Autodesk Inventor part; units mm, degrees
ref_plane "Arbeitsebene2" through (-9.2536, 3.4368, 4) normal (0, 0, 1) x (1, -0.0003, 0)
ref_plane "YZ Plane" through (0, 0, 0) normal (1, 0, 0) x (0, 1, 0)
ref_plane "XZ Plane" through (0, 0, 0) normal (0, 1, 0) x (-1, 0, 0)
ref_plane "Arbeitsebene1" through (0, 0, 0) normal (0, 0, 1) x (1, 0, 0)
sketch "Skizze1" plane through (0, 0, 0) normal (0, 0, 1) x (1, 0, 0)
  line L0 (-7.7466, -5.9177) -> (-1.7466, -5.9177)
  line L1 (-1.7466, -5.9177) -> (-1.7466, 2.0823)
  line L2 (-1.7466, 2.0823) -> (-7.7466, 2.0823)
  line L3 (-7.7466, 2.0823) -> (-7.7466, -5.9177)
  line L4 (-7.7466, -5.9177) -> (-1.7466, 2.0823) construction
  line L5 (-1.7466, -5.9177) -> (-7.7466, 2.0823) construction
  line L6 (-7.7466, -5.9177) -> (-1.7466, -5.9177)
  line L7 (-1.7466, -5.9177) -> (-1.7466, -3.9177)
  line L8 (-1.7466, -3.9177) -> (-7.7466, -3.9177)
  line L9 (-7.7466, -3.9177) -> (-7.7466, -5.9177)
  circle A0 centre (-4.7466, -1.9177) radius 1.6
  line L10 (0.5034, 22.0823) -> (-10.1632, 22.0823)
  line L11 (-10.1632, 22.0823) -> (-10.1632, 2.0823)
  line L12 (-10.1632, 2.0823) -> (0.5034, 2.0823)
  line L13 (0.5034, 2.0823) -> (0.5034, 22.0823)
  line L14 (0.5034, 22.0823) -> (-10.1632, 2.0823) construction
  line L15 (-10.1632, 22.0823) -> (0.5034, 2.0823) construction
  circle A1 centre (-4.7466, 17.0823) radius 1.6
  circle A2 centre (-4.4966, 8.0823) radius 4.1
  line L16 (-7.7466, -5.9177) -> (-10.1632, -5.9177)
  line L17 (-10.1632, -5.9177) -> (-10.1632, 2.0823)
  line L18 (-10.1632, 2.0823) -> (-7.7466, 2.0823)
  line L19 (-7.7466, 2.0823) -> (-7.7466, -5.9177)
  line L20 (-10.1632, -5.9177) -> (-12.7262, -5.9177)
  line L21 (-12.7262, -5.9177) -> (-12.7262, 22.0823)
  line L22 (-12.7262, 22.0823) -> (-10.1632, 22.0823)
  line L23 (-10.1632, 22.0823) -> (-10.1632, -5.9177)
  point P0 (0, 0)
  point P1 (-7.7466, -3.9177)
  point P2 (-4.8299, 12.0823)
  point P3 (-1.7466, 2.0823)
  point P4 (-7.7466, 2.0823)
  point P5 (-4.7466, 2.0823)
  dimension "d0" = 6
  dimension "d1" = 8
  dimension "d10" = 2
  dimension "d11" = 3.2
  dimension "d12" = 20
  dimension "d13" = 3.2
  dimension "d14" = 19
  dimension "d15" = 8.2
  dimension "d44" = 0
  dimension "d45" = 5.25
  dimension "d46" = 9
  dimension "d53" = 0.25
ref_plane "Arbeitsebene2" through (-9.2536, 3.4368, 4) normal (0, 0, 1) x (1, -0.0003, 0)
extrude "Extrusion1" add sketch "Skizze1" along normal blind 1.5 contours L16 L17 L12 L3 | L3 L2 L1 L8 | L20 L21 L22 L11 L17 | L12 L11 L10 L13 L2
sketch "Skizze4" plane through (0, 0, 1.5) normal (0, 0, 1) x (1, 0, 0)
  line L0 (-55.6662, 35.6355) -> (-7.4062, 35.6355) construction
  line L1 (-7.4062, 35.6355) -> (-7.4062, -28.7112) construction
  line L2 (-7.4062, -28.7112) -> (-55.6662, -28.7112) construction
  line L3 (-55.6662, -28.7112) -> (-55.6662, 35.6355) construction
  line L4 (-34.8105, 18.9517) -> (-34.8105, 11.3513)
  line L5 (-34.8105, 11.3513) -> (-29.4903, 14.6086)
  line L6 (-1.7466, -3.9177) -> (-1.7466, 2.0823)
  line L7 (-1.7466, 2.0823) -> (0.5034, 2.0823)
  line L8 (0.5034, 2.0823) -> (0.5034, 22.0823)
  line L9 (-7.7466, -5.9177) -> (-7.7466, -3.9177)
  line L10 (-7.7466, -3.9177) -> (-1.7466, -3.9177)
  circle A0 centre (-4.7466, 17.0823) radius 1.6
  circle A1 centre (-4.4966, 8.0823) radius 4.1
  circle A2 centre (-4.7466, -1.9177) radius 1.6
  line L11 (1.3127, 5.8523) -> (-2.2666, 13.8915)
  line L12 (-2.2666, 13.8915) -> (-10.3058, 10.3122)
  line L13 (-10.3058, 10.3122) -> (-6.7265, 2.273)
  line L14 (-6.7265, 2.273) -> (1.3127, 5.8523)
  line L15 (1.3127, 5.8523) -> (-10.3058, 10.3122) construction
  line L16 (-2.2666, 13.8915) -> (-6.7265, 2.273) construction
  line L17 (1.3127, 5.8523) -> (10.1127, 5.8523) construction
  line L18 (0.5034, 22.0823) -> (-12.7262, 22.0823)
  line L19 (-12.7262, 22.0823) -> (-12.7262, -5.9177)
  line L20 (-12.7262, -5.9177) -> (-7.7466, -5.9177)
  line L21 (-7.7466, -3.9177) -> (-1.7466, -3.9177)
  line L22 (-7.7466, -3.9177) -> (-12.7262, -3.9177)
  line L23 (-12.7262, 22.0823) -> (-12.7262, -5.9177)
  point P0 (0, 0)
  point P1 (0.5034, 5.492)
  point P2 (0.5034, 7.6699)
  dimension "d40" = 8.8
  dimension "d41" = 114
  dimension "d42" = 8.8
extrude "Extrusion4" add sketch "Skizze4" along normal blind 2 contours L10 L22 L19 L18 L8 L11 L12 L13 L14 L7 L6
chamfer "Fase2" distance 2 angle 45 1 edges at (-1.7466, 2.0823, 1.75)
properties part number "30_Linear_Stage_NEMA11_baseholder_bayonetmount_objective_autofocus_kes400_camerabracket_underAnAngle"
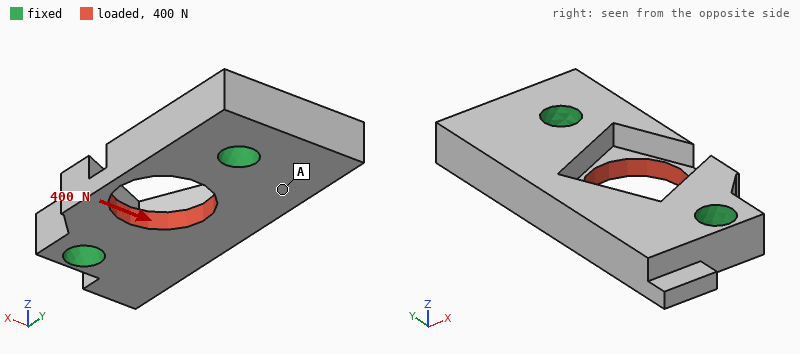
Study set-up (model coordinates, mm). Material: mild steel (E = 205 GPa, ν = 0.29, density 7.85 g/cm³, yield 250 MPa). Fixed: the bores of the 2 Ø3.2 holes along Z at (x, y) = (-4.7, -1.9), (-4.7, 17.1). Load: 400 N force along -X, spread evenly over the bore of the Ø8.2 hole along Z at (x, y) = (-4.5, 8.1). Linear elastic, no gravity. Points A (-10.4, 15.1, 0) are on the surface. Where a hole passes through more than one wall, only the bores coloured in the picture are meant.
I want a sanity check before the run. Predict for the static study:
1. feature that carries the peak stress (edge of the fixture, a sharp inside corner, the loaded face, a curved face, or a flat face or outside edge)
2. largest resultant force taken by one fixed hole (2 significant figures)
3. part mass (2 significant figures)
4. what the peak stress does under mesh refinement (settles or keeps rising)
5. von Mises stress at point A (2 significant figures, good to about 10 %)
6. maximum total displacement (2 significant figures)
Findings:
a sharp inside corner
210 N
7.0 g
keeps rising
7.5 MPa
3.1 µm
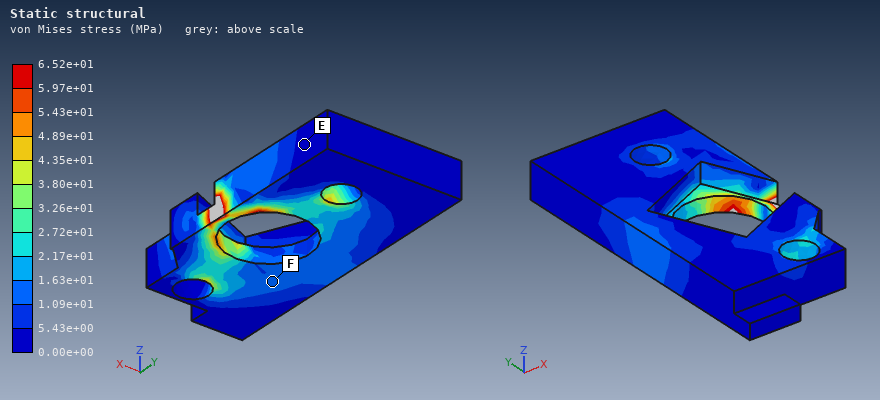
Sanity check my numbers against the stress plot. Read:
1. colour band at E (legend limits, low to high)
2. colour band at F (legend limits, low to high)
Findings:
0.00e+00 to 5.43e+00 MPa
1.09e+01 to 1.63e+01 MPa
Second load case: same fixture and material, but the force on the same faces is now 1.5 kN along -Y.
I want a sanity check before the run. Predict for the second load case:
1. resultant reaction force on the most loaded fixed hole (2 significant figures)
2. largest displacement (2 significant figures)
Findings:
790 N
3.0 µm
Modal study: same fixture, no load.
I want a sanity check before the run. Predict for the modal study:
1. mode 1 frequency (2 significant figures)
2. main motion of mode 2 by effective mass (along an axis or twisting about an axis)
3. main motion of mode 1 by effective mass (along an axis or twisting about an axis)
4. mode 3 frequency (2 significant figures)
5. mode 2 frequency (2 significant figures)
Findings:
32 kHz
twisting about X
along Z
53 kHz
48 kHz
